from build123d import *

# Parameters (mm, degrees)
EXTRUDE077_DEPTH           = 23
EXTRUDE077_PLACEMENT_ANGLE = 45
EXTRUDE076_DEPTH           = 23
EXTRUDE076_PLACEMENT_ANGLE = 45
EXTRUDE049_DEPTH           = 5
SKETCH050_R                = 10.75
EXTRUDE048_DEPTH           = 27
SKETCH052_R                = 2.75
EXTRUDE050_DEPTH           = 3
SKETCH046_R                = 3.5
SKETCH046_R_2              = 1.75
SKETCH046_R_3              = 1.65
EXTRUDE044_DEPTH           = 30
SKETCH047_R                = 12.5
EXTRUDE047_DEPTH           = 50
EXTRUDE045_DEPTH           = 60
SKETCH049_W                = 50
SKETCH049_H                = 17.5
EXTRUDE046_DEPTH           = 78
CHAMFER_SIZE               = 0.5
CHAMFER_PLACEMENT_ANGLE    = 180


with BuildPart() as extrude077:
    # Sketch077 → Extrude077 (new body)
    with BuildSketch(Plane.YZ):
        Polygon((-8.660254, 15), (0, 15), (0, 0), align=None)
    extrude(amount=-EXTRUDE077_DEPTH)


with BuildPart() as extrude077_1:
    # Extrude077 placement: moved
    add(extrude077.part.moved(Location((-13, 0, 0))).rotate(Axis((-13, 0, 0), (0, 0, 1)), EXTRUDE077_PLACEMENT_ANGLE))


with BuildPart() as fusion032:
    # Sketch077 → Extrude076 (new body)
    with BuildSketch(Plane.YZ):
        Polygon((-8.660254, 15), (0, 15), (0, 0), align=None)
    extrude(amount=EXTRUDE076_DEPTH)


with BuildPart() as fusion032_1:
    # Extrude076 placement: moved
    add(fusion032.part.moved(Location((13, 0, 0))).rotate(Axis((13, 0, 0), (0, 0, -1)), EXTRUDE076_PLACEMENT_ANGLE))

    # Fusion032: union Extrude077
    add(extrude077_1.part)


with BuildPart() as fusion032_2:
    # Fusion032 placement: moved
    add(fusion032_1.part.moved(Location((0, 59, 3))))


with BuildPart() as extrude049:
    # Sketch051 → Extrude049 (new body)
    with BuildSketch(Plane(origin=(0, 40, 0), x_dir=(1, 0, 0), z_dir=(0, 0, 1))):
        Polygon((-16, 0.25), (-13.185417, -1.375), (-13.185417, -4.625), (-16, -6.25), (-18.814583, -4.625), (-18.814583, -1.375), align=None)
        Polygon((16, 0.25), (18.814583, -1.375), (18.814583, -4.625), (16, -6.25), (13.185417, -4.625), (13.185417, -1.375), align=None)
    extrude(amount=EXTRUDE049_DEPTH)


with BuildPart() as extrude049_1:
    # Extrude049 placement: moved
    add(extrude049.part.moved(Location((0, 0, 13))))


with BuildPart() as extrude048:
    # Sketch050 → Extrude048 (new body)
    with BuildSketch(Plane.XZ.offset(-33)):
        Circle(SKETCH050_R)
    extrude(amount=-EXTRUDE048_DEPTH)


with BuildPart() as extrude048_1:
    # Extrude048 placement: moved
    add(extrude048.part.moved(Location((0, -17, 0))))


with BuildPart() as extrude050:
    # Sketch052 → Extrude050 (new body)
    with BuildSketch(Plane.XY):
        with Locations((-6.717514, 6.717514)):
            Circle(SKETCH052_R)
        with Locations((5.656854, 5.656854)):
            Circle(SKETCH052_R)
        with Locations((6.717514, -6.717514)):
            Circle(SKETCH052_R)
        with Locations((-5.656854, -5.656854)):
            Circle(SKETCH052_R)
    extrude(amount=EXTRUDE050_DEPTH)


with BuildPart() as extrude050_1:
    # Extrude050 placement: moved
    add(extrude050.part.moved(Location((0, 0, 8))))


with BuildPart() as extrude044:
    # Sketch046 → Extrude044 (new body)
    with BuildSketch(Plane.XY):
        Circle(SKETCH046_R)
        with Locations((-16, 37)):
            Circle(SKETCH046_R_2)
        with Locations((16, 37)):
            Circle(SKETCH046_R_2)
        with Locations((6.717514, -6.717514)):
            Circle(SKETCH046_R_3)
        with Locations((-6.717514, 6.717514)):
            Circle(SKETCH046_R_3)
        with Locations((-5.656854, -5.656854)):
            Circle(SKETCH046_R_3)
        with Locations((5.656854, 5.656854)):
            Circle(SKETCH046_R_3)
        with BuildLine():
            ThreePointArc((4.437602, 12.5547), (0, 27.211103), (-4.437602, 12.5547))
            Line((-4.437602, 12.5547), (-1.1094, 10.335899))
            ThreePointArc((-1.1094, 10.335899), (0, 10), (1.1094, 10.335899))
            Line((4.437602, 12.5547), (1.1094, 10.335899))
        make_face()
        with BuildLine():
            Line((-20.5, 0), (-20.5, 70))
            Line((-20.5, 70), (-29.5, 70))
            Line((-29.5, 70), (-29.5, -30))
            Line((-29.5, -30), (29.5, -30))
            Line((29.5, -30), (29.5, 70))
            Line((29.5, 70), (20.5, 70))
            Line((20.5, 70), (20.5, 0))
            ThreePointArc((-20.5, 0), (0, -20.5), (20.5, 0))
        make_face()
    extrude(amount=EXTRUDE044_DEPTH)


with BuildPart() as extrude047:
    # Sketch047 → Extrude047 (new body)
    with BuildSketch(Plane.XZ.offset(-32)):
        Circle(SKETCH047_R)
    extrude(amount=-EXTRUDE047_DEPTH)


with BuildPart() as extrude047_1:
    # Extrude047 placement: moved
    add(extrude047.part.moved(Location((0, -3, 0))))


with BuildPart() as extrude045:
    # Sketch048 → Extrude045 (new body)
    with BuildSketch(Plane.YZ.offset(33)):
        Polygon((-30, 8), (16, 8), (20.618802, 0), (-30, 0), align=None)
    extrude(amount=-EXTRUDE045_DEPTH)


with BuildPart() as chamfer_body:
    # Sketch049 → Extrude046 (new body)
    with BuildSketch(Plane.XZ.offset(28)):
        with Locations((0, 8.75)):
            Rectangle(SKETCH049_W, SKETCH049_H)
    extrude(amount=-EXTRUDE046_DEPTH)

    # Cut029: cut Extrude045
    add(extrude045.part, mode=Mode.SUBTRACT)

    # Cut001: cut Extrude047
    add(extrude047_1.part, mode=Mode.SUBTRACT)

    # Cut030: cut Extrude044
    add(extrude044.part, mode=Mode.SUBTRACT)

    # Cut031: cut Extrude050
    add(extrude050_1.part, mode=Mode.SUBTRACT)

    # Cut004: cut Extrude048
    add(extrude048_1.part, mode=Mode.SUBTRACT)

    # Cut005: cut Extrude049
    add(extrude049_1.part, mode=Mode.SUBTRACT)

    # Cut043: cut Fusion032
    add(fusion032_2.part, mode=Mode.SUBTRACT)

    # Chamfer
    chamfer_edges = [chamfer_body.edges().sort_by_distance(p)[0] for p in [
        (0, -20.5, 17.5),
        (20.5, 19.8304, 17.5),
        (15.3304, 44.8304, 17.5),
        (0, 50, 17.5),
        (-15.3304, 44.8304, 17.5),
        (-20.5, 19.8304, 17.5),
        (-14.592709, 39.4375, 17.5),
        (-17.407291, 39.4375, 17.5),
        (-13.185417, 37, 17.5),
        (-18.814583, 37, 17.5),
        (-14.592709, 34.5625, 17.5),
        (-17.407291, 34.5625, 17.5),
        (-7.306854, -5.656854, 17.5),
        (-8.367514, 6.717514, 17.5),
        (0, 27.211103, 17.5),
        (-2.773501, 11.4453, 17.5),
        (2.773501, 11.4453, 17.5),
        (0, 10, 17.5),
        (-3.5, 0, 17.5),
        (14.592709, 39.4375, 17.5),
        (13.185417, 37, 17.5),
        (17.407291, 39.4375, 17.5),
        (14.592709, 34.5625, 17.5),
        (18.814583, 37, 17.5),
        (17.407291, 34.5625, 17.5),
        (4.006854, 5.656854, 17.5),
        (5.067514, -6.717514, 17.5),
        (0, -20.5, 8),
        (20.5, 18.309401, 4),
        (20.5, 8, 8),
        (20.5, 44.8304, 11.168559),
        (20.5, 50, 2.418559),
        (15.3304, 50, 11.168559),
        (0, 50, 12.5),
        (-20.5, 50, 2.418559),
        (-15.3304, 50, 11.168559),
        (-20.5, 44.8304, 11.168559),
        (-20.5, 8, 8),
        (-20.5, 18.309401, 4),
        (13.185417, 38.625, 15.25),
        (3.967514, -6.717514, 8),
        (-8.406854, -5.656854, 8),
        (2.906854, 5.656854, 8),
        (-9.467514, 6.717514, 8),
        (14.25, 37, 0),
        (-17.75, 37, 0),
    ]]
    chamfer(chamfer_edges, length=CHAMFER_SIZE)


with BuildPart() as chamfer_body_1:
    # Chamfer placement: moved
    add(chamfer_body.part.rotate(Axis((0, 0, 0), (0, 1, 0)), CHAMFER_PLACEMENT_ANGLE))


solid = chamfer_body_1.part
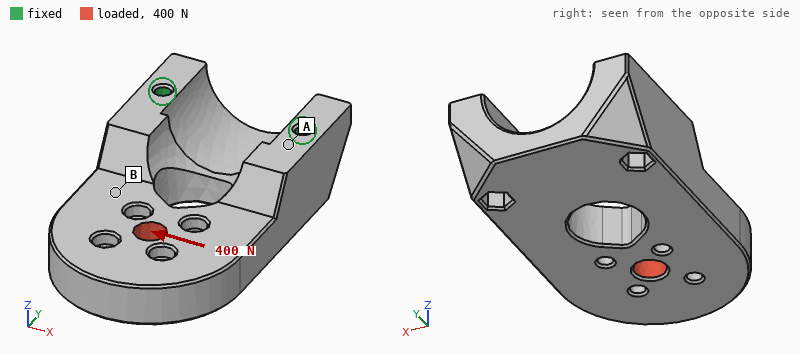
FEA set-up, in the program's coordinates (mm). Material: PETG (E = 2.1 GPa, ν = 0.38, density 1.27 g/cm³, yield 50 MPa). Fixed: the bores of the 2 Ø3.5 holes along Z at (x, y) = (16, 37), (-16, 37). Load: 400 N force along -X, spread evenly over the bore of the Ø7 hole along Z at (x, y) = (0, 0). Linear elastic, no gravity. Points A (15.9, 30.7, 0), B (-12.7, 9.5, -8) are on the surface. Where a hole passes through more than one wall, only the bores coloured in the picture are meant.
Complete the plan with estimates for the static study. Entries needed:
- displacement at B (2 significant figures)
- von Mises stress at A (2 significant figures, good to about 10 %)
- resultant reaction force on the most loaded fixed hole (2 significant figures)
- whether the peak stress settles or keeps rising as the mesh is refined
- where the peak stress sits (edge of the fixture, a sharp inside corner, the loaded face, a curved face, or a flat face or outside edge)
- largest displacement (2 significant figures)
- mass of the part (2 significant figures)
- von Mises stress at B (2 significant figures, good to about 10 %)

0.17 mm
1.6 MPa
460 N
keeps rising
edge of the fixture
0.27 mm
32 g
3.4 MPa
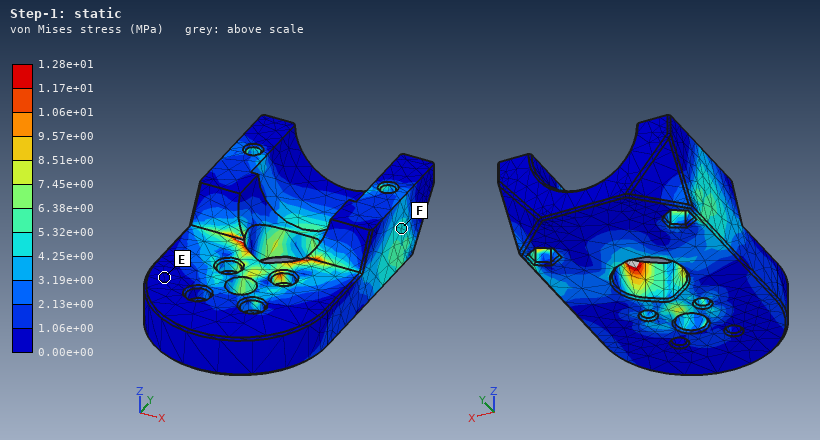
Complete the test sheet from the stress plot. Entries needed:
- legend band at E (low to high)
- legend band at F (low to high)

0.00e+00 to 1.06e+00 MPa
4.25e+00 to 5.32e+00 MPa
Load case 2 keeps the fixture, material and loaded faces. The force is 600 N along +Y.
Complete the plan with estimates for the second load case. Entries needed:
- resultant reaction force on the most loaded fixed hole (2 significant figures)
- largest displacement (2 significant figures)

300 N
0.15 mm
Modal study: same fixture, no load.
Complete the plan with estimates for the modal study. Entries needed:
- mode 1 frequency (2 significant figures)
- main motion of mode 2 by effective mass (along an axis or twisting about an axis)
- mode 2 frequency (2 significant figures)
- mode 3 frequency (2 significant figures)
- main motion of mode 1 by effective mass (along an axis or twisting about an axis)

820 Hz
along X
1700 Hz
2300 Hz
along Z
